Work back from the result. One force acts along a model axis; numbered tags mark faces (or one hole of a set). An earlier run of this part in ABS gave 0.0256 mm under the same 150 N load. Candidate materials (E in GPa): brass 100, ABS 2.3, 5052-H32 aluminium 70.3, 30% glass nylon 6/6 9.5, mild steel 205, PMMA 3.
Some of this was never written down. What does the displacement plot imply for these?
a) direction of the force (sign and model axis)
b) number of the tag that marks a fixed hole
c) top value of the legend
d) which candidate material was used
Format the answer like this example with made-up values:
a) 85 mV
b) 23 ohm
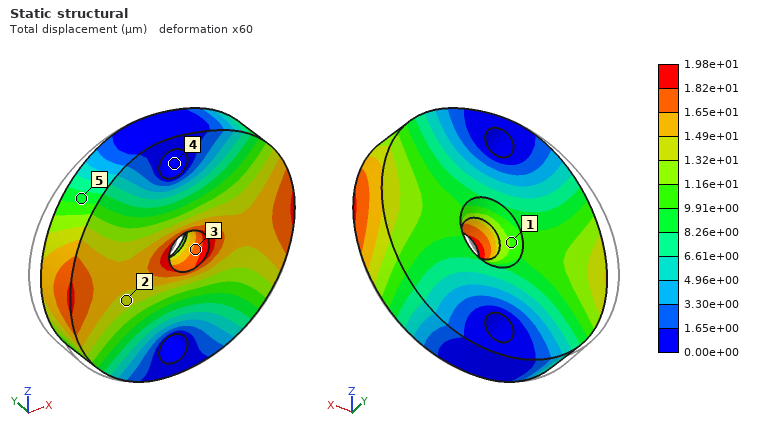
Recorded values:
a) +X
b) 4
c) 1.98e+01 µm
d) PMMA
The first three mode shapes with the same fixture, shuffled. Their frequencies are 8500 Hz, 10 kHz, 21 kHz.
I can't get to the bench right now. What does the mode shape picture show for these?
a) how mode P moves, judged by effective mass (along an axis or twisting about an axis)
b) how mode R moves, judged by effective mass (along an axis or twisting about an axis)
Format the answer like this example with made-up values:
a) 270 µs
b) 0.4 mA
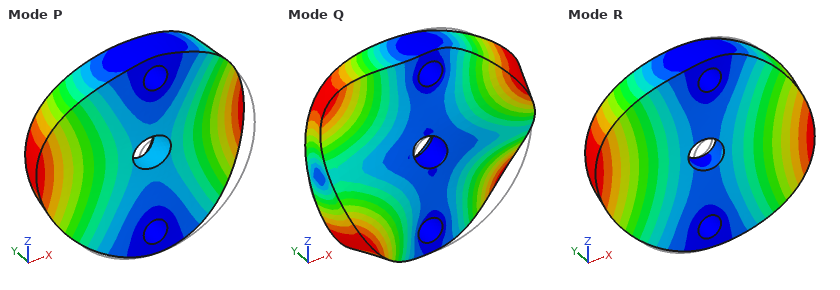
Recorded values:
a) along Y
b) twisting about Z
